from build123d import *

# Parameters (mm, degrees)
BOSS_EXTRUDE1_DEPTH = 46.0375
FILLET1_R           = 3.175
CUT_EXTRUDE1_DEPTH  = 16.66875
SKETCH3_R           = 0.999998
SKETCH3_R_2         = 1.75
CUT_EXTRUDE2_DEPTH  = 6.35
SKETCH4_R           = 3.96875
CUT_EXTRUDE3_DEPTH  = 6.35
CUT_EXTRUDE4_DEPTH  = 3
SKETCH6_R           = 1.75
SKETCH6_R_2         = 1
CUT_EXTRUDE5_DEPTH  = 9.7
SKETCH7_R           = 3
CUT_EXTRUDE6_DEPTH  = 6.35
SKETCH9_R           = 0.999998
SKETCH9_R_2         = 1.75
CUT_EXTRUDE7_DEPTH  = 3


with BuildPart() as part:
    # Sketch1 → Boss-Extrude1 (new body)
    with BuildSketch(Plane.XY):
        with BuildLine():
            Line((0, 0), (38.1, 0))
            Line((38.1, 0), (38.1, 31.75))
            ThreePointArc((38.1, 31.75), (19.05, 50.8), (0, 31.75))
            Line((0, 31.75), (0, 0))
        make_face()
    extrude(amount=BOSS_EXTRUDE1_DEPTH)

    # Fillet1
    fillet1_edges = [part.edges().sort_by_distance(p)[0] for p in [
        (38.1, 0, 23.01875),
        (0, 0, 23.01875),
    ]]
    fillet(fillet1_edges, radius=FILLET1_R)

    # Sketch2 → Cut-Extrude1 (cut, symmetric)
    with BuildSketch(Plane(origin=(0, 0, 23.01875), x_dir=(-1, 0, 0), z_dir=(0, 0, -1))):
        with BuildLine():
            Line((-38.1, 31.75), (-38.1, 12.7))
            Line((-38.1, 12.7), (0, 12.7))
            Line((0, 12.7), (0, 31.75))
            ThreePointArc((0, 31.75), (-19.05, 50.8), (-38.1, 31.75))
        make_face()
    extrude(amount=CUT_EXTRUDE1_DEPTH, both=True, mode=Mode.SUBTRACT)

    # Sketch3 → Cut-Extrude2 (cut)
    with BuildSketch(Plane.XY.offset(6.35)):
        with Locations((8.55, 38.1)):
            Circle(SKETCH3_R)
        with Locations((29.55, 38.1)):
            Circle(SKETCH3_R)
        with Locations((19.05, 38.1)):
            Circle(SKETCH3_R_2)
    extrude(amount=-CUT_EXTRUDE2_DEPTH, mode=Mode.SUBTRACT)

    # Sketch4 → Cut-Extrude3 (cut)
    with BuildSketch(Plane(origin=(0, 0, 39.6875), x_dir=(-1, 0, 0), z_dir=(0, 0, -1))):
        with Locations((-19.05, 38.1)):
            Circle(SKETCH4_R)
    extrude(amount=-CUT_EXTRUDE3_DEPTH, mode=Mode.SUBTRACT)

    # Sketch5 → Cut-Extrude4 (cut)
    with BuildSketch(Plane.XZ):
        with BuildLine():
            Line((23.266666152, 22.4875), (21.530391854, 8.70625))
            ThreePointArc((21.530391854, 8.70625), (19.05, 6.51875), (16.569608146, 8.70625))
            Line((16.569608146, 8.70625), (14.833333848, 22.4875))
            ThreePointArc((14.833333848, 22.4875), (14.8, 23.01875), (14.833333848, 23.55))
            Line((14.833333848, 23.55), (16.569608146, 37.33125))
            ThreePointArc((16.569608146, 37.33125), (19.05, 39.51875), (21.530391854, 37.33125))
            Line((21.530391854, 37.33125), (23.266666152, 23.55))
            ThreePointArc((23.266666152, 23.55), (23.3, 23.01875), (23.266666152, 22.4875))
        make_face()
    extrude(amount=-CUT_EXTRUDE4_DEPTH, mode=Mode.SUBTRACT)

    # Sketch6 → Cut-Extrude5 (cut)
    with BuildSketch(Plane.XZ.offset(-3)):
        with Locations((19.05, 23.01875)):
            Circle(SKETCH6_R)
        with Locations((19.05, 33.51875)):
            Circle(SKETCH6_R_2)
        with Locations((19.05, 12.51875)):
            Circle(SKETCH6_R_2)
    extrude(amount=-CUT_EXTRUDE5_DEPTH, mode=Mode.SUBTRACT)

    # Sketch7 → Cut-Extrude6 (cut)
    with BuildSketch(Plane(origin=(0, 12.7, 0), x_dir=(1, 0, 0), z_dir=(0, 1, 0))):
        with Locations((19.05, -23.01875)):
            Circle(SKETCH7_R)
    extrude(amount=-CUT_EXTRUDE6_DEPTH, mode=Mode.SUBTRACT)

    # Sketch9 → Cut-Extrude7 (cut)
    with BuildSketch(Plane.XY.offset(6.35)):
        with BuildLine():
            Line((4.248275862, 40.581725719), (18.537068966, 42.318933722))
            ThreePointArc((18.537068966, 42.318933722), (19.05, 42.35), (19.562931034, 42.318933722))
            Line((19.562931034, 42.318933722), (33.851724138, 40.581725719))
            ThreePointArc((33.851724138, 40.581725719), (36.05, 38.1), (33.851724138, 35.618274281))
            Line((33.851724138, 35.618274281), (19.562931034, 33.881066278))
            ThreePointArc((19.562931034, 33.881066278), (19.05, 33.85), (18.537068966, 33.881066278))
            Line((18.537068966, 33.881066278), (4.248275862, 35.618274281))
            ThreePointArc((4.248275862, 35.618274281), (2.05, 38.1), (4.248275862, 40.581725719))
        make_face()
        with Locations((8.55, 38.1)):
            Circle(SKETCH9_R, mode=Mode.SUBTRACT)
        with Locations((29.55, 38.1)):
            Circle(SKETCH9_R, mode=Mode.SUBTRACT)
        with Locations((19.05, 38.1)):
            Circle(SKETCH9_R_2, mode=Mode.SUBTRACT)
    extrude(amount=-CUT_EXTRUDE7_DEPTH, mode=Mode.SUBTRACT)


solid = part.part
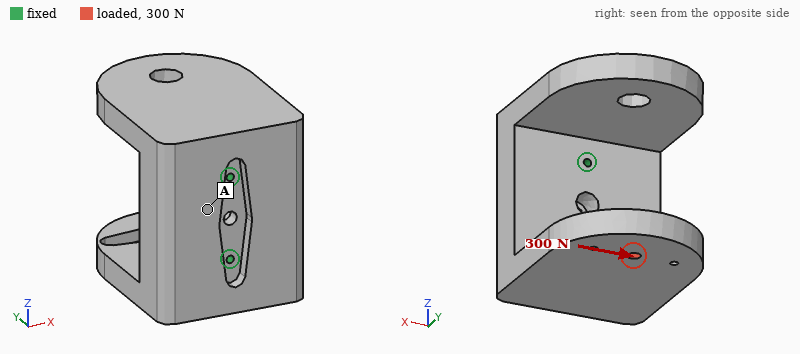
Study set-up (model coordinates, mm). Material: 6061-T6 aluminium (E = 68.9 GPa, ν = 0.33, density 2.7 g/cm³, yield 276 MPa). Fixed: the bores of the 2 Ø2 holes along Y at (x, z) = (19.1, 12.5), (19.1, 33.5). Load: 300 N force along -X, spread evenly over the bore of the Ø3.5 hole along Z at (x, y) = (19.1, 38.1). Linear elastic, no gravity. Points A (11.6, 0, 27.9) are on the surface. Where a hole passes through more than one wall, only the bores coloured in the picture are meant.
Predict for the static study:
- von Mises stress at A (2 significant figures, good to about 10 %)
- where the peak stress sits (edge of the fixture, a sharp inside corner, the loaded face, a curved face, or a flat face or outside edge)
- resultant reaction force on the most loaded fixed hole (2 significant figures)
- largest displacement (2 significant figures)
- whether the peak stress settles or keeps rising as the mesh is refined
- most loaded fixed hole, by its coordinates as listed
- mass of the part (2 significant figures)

4.1 MPa
edge of the fixture
450 N
27 µm
keeps rising
(19.1, 12.5)
99 g
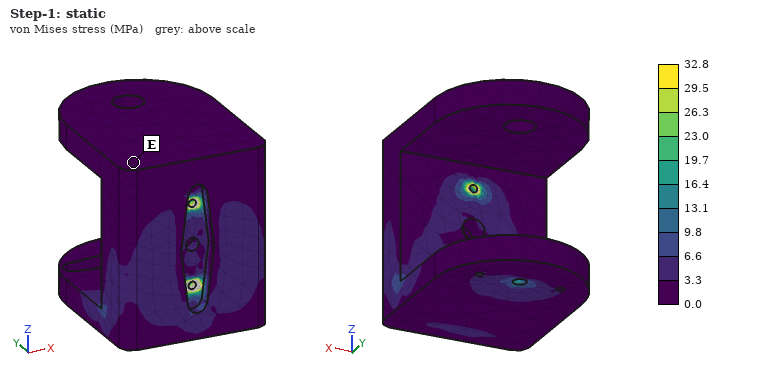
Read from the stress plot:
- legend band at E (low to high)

0.0 to 3.3 MPa
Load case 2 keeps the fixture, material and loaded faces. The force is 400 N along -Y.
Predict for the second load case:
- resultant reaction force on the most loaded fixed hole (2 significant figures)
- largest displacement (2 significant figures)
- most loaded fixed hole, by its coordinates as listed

510 N
16 µm
(19.1, 12.5)
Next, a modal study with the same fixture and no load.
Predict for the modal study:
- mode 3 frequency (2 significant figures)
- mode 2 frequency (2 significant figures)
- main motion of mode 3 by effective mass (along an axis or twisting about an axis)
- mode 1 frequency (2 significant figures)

4100 Hz
3400 Hz
along X
3300 Hz
